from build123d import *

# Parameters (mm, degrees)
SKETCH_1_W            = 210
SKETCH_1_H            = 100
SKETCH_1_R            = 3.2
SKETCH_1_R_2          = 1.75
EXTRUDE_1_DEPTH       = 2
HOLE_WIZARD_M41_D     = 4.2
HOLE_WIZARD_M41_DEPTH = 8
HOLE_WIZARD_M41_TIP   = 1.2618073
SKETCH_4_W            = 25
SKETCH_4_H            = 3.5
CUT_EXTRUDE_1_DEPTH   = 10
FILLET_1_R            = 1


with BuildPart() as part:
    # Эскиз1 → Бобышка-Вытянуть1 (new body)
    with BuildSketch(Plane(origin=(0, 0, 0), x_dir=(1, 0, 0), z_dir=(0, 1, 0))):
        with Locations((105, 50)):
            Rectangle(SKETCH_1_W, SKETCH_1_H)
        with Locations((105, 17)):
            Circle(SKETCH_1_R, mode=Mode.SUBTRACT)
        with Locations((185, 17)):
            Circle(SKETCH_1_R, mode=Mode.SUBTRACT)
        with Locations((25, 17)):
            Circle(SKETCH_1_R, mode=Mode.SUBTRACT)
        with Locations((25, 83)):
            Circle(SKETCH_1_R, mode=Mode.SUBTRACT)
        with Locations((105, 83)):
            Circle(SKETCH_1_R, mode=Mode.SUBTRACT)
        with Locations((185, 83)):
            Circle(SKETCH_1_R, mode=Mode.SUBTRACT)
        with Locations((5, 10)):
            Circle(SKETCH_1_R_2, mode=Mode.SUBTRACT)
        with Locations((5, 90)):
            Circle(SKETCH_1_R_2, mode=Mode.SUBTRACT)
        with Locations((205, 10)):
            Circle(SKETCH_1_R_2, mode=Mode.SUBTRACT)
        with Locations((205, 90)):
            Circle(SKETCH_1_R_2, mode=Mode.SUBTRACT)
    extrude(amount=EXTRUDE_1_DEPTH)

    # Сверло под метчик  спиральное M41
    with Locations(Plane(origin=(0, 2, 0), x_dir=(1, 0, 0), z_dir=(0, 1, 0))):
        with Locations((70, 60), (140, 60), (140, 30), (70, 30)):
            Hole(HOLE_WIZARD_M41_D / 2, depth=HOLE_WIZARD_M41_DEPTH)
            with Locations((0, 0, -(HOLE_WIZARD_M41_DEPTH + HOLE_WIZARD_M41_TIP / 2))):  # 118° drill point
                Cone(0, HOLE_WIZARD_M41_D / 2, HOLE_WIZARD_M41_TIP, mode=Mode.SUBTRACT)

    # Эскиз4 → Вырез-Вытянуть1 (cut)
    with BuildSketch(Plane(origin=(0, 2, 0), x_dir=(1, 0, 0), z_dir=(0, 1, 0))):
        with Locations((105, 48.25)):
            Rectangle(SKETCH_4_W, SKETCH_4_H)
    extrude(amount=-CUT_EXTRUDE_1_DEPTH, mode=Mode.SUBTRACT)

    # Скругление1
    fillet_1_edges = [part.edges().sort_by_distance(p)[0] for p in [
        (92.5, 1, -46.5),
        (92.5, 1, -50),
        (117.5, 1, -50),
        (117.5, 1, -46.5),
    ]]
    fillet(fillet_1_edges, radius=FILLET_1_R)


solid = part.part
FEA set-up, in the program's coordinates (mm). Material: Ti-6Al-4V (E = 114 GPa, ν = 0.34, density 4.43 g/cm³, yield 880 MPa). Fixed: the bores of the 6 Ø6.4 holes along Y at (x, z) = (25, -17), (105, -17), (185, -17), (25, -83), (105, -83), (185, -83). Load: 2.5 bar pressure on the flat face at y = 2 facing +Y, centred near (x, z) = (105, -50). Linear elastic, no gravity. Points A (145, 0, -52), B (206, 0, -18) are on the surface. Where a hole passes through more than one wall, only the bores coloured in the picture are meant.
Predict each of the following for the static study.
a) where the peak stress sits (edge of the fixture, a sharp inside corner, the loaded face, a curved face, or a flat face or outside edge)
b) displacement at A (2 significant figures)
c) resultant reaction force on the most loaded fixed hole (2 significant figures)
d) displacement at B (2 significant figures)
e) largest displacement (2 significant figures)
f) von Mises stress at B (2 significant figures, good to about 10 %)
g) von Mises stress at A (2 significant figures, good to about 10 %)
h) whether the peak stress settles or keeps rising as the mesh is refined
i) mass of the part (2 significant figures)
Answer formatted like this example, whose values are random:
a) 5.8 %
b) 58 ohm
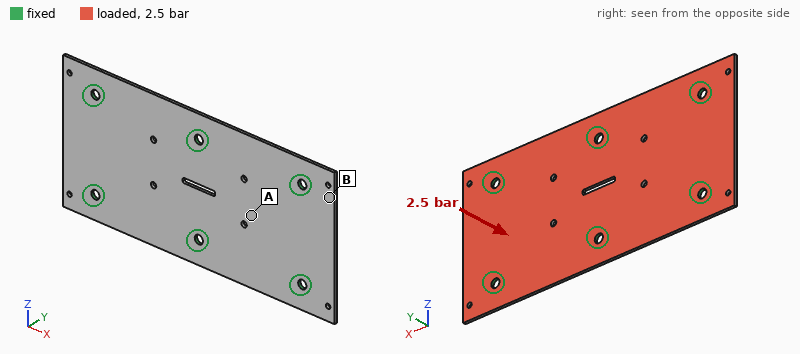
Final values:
a) edge of the fixture
b) 0.46 mm
c) 990 N
d) 0.085 mm
e) 0.46 mm
f) 28 MPa
g) 84 MPa
h) keeps rising
i) 180 g
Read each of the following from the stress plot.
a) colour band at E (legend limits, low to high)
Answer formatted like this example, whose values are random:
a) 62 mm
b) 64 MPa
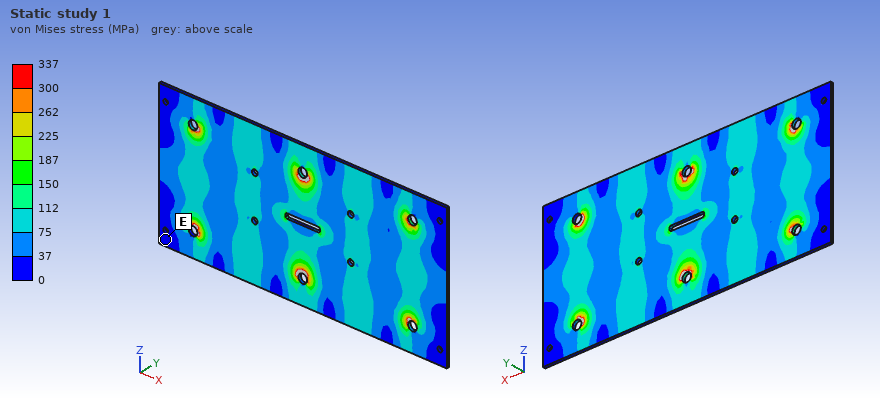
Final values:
a) 0 to 37 MPa
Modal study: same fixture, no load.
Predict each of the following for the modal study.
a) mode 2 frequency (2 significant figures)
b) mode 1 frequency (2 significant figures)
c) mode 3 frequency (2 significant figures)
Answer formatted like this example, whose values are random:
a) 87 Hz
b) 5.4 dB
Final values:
a) 1500 Hz
b) 1400 Hz
c) 1800 Hz
